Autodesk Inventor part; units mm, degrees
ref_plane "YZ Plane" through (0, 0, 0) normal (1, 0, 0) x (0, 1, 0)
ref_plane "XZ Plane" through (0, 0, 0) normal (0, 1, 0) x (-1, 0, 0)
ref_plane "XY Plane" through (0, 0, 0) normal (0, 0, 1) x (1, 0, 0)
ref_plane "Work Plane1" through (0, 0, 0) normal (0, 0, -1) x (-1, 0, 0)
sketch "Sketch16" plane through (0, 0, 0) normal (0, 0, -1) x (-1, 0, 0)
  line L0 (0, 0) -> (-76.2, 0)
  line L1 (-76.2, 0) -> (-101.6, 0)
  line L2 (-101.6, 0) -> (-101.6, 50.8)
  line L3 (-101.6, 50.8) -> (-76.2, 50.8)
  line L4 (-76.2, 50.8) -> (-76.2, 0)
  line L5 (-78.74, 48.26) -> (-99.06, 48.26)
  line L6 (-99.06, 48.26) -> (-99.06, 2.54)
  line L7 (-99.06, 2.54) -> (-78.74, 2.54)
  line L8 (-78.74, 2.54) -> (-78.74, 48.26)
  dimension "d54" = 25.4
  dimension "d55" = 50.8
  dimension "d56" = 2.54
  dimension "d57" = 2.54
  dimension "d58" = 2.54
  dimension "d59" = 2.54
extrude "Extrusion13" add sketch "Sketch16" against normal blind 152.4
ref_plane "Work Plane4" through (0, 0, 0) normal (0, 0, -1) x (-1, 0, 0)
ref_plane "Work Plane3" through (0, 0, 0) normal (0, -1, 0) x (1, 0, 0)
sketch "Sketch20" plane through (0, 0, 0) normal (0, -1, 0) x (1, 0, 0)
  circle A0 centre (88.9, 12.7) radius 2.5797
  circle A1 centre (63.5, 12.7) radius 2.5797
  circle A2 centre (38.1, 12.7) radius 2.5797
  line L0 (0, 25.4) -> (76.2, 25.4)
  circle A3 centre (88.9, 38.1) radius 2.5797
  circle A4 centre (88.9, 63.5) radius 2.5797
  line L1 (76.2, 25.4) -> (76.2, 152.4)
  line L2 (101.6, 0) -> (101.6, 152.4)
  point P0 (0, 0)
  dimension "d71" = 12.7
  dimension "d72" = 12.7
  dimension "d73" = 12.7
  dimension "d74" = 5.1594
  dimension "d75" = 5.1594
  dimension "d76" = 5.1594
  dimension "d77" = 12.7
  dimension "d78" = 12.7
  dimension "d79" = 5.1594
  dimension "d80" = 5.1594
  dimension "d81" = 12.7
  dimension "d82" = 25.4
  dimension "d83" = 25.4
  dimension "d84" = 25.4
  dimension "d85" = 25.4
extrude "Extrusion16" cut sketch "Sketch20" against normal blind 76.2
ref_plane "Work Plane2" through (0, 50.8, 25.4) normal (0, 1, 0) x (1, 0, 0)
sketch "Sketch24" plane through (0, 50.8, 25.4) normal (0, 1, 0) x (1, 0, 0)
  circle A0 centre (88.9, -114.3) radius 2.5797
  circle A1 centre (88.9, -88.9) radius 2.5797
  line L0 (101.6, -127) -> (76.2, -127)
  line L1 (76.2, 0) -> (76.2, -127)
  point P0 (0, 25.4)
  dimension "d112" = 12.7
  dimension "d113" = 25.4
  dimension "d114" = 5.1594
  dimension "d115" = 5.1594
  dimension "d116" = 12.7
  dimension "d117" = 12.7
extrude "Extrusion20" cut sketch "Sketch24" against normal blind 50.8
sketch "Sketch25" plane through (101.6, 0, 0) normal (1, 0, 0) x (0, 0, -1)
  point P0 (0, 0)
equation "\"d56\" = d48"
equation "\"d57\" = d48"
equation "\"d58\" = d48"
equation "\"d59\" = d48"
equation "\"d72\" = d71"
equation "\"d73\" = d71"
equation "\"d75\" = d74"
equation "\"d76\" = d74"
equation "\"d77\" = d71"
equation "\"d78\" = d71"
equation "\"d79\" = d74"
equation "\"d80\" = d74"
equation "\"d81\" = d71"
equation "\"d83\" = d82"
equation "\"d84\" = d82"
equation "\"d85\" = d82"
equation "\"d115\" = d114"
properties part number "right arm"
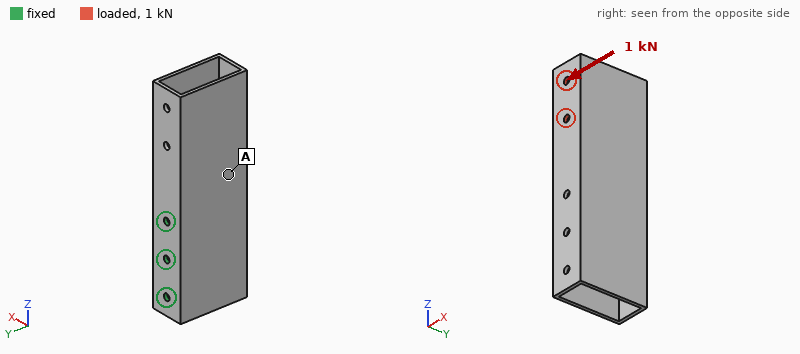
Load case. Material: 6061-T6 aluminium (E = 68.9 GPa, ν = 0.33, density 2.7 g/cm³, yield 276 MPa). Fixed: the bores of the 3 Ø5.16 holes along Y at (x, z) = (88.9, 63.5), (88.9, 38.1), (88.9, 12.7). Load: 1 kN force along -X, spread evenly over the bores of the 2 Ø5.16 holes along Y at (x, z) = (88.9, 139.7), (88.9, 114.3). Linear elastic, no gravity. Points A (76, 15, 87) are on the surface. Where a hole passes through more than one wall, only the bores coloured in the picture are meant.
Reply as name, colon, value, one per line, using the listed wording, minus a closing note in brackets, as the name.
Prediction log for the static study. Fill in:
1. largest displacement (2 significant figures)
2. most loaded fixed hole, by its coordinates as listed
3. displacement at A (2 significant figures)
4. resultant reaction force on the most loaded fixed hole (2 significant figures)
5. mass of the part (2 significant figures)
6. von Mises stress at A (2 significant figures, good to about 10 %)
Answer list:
largest displacement: 1.5 mm
most loaded fixed hole, by its coordinates as listed: (88.9, 63.5)
displacement at A: 0.99 mm
resultant reaction force on the most loaded fixed hole: 2.3 kN
mass of the part: 150 g
von Mises stress at A: 42 MPa
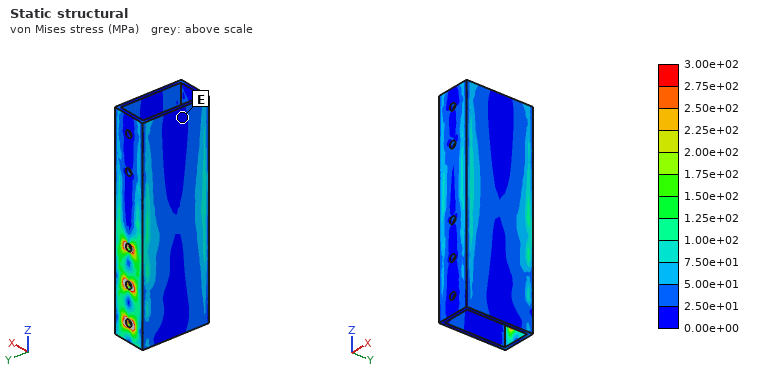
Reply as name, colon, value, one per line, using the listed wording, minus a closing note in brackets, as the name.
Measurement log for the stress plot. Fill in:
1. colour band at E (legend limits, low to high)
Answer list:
colour band at E: 0.00e+00 to 2.50e+01 MPa
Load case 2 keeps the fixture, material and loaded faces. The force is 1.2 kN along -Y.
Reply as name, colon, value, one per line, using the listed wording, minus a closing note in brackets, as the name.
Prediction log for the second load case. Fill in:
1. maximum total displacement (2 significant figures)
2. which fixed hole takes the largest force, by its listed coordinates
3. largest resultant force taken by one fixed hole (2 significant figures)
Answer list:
maximum total displacement: 0.53 mm
which fixed hole takes the largest force, by its listed coordinates: (88.9, 63.5)
largest resultant force taken by one fixed hole: 2.5 kN
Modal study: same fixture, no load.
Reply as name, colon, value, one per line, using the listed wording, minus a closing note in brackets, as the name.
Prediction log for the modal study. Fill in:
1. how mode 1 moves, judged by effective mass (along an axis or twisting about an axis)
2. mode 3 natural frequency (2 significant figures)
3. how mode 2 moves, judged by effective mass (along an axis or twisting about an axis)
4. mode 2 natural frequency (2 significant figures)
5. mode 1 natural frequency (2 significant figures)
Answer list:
how mode 1 moves, judged by effective mass: along X
mode 3 natural frequency: 1400 Hz
how mode 2 moves, judged by effective mass: along Y
mode 2 natural frequency: 1100 Hz
mode 1 natural frequency: 560 Hz
